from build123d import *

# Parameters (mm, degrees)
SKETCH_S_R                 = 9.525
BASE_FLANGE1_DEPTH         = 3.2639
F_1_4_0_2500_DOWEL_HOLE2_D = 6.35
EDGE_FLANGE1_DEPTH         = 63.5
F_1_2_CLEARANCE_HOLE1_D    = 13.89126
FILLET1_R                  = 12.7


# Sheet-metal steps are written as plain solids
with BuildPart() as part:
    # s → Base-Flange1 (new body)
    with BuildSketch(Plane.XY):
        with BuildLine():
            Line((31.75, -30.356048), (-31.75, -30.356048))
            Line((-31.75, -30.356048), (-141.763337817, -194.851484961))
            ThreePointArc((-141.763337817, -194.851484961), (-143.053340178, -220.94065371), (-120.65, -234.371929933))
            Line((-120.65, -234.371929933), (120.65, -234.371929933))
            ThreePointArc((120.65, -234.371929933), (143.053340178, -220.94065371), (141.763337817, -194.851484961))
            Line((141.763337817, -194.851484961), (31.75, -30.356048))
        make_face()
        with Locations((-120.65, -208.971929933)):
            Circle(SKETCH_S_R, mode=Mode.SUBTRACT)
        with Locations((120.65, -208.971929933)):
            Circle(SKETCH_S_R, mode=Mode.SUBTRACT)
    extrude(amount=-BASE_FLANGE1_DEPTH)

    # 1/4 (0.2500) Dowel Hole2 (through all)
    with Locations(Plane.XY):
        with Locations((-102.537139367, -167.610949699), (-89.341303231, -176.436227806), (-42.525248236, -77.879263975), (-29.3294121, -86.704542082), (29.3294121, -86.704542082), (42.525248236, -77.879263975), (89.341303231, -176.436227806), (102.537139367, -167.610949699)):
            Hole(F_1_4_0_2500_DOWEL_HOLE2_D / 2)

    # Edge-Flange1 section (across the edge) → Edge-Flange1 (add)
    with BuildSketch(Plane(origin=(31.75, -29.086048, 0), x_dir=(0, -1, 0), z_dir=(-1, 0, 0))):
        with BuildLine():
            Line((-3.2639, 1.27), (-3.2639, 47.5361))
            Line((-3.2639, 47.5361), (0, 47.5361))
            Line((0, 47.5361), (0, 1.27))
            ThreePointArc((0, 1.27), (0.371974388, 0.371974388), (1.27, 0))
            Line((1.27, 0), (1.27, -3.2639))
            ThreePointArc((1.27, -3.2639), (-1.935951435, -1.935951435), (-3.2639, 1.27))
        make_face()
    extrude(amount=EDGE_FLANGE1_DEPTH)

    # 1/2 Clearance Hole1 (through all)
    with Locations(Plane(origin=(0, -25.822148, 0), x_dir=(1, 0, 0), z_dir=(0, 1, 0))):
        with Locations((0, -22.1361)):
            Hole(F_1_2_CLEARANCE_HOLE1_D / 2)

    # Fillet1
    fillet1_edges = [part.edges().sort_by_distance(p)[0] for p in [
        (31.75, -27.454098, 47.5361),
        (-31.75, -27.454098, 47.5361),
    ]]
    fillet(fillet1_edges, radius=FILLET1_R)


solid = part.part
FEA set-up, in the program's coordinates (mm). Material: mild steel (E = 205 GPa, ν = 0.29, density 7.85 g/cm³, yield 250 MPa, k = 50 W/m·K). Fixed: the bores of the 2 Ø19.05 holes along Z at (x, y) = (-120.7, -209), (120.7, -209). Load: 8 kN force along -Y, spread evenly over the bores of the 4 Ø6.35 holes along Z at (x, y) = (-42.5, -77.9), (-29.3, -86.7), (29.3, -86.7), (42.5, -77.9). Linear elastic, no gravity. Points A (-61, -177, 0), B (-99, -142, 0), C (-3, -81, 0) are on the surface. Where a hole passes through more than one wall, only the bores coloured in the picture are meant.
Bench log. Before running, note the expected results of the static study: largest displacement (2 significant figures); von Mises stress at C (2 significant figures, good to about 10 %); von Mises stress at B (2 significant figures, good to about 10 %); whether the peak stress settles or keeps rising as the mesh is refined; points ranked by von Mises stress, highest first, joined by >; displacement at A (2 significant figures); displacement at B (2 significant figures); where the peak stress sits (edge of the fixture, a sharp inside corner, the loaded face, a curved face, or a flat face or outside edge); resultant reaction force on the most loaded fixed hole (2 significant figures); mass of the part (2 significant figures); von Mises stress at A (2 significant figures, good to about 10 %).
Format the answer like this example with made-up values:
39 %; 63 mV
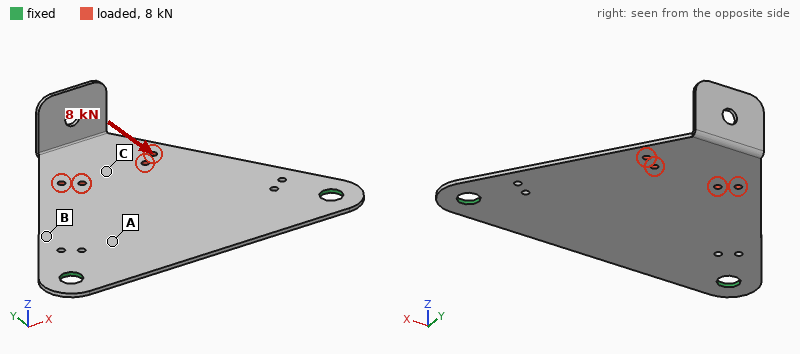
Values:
22 µm; 6.7 MPa; 25 MPa; keeps rising; B > A > C; 13 µm; 9.5 µm; edge of the fixture; 4.6 kN; 1.1 kg; 16 MPa
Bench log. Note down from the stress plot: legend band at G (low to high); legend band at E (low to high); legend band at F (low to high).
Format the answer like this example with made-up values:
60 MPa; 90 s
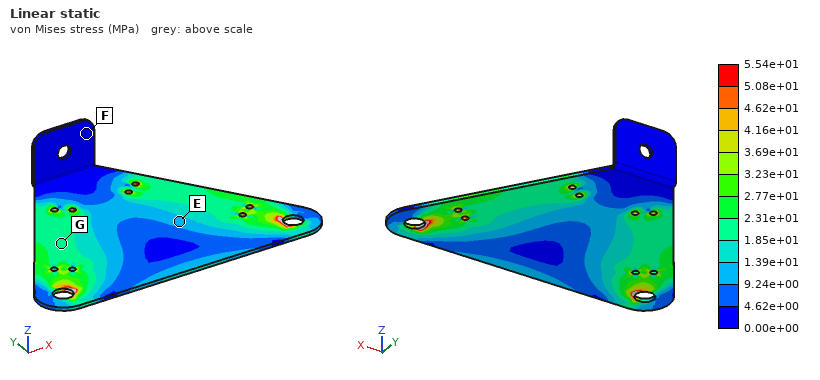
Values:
1.85e+01 to 2.31e+01 MPa; 9.24e+00 to 1.39e+01 MPa; 0.00e+00 to 4.62e+00 MPa
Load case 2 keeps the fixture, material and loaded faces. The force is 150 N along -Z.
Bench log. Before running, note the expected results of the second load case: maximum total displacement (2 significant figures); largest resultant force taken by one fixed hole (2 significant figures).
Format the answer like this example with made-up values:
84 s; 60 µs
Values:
2.1 mm; 75 N
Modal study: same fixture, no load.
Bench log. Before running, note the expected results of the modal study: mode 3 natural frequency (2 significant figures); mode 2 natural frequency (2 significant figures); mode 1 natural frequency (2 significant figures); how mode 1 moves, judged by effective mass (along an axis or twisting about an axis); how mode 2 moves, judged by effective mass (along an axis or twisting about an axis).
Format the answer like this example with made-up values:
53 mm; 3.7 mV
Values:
310 Hz; 290 Hz; 74 Hz; along Z; along Z
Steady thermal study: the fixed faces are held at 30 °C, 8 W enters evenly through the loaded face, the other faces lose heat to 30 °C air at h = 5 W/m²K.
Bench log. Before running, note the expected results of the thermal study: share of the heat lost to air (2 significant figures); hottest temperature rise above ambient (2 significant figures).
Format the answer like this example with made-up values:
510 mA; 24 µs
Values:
63 %; 27 K
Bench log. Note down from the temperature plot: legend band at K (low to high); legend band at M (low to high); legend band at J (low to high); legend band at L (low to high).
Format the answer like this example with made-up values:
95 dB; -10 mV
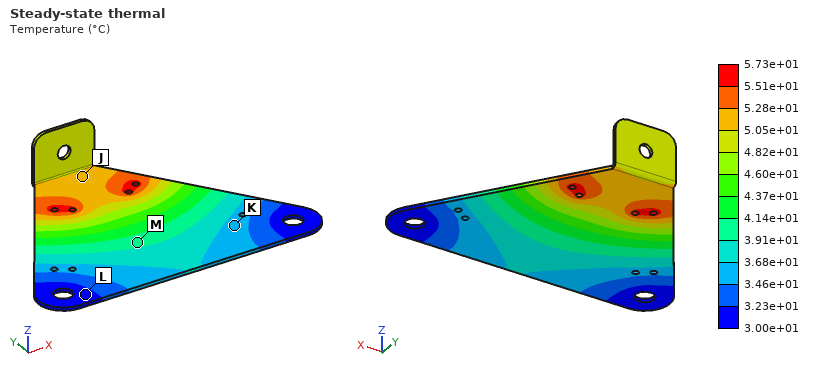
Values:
3.46e+01 to 3.68e+01 °C; 3.91e+01 to 4.14e+01 °C; 5.05e+01 to 5.28e+01 °C; 3.00e+01 to 3.23e+01 °C
